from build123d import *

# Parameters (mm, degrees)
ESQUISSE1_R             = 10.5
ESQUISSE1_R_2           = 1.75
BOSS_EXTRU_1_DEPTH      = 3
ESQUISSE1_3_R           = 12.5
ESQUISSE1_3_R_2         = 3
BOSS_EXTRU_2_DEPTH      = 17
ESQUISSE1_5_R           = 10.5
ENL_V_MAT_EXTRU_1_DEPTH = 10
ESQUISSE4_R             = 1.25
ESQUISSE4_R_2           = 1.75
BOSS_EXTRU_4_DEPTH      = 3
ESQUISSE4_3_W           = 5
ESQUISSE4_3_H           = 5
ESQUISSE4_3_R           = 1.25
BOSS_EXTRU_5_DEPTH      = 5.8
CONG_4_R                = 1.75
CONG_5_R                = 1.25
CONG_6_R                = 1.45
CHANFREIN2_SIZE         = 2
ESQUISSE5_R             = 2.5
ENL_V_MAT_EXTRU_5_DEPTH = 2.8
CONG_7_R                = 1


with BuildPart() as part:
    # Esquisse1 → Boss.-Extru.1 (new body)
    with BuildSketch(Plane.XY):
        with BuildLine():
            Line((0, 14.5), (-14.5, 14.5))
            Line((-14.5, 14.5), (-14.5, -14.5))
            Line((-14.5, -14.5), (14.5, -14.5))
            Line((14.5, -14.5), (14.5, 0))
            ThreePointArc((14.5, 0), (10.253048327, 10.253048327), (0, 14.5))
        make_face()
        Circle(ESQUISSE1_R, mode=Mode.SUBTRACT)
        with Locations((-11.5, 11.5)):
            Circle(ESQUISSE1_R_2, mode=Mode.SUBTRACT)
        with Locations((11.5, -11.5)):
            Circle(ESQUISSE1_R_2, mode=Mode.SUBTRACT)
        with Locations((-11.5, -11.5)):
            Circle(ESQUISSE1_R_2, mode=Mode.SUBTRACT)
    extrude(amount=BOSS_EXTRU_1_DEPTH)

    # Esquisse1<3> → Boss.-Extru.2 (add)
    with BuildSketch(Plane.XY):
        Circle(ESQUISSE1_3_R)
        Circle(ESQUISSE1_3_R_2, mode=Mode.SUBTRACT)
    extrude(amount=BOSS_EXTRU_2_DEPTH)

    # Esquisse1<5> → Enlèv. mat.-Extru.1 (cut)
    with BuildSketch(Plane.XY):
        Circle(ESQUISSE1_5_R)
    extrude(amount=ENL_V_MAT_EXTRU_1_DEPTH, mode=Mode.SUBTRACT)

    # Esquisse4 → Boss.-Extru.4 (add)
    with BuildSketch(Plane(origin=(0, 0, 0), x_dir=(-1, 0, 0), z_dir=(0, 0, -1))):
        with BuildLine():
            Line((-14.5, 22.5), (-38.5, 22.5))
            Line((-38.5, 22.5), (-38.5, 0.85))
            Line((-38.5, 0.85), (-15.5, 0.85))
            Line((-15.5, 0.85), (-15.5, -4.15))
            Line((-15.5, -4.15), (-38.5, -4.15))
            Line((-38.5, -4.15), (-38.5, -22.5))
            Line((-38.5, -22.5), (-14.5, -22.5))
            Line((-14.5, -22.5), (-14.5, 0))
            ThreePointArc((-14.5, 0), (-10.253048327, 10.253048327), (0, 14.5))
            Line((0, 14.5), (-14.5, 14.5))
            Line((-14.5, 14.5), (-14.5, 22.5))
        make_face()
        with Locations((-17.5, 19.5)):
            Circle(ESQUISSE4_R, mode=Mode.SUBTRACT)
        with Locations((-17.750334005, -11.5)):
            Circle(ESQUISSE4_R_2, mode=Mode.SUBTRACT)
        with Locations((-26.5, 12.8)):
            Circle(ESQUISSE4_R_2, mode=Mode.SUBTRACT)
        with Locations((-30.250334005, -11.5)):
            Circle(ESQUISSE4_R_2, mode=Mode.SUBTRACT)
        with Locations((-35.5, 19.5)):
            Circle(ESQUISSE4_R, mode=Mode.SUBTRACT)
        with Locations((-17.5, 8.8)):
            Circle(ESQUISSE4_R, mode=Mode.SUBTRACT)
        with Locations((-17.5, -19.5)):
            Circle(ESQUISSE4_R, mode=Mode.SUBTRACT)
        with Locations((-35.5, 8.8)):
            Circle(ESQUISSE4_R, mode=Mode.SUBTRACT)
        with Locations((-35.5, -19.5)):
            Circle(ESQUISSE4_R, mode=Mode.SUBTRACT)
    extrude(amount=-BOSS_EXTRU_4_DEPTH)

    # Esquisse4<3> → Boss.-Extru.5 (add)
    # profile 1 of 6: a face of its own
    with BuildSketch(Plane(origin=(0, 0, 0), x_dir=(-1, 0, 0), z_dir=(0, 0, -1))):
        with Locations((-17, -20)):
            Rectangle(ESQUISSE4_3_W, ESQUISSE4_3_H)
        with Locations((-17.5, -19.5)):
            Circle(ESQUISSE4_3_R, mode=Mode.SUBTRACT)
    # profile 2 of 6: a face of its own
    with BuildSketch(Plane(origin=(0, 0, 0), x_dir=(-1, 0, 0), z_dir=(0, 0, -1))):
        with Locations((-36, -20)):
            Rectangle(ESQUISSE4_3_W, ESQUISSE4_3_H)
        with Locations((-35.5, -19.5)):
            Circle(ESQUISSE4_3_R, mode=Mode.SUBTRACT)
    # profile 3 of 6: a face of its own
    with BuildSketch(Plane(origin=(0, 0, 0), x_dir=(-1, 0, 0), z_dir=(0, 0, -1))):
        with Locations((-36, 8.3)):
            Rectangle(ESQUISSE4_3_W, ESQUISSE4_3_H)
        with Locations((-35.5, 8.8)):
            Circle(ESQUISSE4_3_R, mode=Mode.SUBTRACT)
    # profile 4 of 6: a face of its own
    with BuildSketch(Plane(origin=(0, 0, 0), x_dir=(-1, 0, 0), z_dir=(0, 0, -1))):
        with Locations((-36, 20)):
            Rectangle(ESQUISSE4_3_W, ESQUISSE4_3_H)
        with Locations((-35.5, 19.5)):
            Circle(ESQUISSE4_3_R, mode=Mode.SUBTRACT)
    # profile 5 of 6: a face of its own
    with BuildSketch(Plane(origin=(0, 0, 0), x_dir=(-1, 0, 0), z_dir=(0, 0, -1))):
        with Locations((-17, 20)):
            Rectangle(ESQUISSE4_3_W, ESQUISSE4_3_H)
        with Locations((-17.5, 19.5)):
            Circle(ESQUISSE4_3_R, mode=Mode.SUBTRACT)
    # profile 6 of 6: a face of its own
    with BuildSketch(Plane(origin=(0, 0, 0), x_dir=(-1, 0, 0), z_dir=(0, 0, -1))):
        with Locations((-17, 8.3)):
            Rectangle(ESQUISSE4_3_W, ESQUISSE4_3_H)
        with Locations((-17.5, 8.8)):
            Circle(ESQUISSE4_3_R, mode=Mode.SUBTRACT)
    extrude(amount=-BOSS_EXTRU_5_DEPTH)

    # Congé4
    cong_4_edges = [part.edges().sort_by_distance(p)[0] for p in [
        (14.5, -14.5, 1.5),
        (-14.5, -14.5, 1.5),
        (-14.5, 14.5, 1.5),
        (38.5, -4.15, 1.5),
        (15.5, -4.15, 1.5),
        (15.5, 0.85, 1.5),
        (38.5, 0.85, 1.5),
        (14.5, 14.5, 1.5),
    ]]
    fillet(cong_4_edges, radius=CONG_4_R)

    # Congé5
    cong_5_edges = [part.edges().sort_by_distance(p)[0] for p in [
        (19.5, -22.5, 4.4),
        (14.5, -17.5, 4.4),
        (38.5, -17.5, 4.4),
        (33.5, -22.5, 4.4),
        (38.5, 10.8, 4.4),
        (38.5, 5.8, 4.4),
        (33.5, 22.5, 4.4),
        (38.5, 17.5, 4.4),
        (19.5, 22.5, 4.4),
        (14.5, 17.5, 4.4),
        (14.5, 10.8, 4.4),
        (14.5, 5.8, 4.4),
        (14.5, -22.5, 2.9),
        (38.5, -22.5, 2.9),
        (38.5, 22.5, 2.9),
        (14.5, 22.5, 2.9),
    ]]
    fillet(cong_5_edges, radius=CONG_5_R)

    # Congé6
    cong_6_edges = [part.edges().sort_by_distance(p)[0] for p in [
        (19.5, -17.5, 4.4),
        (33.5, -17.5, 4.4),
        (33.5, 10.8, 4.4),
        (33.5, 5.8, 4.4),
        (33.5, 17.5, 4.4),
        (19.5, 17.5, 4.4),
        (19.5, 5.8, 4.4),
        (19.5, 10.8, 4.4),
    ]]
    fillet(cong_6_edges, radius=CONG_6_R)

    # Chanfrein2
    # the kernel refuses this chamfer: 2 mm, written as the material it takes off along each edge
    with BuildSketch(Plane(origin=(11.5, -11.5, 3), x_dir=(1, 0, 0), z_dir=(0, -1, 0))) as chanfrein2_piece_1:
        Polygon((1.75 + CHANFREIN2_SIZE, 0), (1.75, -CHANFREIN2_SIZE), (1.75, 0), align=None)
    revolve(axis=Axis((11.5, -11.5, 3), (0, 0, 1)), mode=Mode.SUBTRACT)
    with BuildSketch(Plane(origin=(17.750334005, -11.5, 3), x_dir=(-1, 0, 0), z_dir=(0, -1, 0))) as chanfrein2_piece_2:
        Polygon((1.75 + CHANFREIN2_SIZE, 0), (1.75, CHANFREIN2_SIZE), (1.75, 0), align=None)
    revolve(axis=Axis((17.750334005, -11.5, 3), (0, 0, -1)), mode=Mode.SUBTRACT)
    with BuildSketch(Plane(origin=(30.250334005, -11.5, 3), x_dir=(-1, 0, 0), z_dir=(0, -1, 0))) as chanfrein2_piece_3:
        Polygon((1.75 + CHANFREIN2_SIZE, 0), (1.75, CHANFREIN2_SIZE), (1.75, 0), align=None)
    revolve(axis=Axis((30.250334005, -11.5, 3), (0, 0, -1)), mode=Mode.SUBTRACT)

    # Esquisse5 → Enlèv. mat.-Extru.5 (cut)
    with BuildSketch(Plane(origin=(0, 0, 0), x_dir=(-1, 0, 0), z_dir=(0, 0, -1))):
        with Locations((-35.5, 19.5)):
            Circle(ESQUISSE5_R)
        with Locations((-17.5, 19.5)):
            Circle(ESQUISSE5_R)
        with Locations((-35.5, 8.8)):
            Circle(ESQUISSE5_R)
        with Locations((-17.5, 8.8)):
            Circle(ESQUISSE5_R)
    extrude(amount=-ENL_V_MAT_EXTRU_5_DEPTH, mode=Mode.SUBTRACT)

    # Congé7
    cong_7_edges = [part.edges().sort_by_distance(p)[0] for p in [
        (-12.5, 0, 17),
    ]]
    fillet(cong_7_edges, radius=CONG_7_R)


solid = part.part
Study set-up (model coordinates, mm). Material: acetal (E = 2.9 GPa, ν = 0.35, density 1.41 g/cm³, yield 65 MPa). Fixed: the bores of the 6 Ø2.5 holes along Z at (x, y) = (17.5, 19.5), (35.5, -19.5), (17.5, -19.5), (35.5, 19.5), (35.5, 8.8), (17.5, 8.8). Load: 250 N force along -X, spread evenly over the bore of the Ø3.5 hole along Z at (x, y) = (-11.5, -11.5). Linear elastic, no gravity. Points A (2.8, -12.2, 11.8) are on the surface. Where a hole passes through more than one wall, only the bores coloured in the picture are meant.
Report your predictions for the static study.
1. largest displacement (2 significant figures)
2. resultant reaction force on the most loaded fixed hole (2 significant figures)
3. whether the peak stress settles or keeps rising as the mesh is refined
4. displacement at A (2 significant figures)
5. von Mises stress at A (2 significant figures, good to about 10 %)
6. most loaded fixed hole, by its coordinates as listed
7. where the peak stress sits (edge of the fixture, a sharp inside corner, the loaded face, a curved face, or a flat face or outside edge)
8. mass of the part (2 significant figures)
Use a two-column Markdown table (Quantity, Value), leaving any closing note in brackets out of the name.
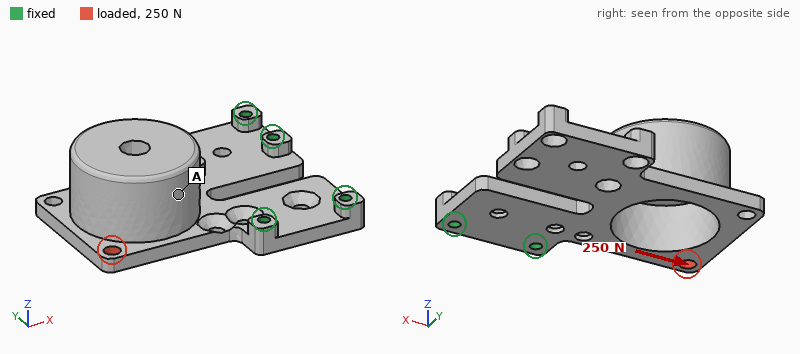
| Quantity | Value |
|---|---|
| largest displacement | 0.35 mm |
| resultant reaction force on the most loaded fixed hole | 150 N |
| whether the peak stress settles or keeps rising as the mesh is refined | keeps rising |
| displacement at A | 0.21 mm |
| von Mises stress at A | 3.5 MPa |
| most loaded fixed hole, by its coordinates as listed | (17.5, -19.5) |
| where the peak stress sits | a sharp inside corner |
| mass of the part | 12 g |
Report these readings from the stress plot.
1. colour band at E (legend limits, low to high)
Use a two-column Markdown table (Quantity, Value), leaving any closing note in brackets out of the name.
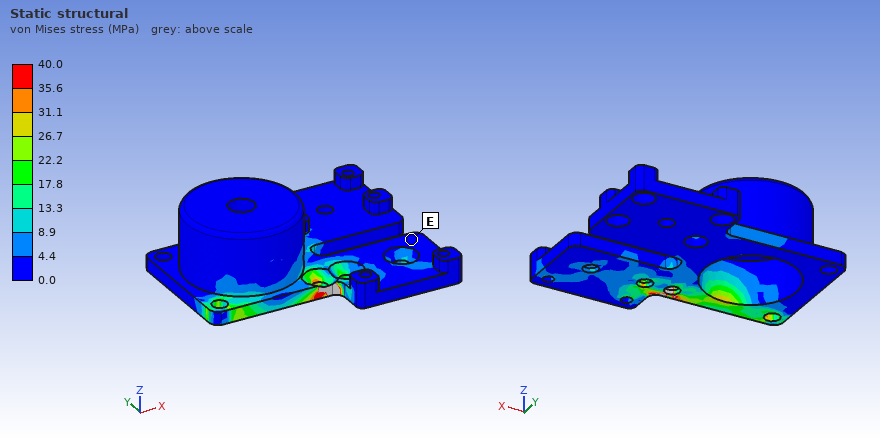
| Quantity | Value |
|---|---|
| colour band at E | 0.0 to 4.4 MPa |
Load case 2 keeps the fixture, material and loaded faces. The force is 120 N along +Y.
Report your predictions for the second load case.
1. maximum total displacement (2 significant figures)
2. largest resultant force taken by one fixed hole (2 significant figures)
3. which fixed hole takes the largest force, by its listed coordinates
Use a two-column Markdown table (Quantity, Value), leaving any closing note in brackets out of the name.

| Quantity | Value |
|---|---|
| maximum total displacement | 0.66 mm |
| largest resultant force taken by one fixed hole | 84 N |
| which fixed hole takes the largest force, by its listed coordinates | (17.5, -19.5) |
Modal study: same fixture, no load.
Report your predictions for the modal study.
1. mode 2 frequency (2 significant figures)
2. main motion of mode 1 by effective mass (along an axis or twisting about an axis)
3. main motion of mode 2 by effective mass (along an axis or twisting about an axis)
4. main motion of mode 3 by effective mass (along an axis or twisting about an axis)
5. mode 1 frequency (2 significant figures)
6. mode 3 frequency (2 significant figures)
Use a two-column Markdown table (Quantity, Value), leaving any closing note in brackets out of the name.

| Quantity | Value |
|---|---|
| mode 2 frequency | 1100 Hz |
| main motion of mode 1 by effective mass | along Z |
| main motion of mode 2 by effective mass | along Y |
| main motion of mode 3 by effective mass | along Y |
| mode 1 frequency | 360 Hz |
| mode 3 frequency | 1800 Hz |
